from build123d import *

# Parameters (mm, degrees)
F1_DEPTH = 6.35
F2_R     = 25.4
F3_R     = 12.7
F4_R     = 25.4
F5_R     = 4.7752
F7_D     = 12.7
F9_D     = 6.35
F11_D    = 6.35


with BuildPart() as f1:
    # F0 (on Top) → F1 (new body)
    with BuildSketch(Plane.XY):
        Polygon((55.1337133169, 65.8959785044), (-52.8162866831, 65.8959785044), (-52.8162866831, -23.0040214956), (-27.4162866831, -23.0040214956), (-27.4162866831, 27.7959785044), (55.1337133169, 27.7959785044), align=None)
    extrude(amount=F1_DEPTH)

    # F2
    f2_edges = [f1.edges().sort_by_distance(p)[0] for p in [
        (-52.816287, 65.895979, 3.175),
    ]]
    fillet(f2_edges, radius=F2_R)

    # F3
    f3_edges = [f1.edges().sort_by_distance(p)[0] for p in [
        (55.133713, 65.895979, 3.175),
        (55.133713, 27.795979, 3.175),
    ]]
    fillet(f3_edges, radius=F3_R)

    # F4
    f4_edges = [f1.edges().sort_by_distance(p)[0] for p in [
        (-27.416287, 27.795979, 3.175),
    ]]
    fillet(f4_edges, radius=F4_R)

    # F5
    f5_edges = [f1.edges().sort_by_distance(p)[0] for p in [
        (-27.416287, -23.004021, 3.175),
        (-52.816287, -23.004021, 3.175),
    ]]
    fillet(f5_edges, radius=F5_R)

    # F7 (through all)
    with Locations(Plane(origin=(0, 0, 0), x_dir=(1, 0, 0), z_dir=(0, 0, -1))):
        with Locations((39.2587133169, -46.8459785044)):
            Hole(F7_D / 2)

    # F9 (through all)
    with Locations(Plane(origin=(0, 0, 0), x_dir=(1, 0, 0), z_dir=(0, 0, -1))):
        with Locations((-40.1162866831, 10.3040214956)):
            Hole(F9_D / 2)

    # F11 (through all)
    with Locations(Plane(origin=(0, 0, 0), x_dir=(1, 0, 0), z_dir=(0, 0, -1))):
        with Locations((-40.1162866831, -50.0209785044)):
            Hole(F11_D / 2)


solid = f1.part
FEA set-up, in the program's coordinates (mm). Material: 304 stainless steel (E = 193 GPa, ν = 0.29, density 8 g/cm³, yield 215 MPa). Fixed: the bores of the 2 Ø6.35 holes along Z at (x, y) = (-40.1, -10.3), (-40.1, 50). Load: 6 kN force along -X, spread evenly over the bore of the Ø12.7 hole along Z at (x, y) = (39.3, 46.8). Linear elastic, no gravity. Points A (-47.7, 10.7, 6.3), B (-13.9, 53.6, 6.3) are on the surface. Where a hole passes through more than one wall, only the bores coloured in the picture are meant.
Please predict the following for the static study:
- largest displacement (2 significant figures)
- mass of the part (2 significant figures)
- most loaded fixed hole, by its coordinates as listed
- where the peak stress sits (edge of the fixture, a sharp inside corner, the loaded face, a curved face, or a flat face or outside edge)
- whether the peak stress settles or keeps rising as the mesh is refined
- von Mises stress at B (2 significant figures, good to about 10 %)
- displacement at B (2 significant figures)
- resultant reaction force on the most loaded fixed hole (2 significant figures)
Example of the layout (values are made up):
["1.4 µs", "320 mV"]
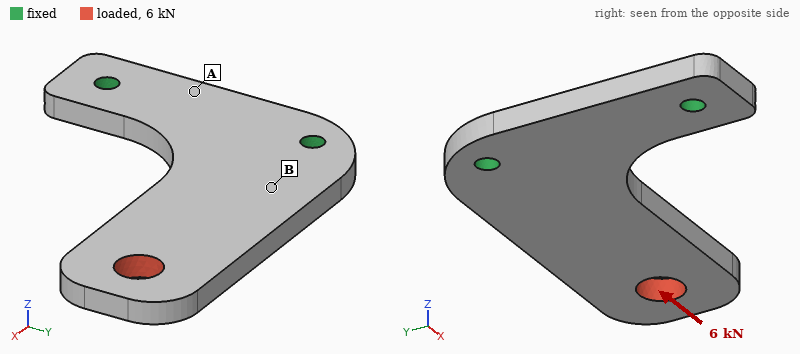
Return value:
["15 µm", "260 g", "(-40.1, 50)", "edge of the fixture", "keeps rising", "27 MPa", "5.1 µm", "5.6 kN"]
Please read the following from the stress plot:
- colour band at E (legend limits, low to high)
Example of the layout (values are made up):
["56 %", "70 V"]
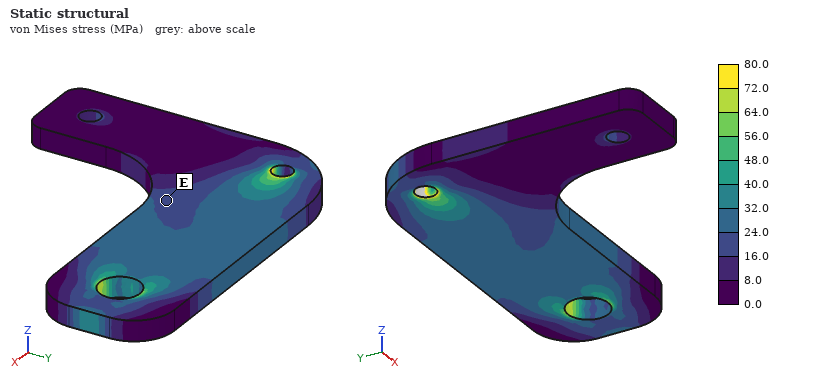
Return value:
["16.0 to 24.0 MPa"]
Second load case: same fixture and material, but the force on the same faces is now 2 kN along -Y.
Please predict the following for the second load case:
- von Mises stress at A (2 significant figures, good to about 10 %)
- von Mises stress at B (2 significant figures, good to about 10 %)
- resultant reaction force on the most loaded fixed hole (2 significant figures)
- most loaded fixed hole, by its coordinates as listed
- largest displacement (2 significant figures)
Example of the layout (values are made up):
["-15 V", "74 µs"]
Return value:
["22 MPa", "27 MPa", "3.1 kN", "(-40.1, -10.3)", "91 µm"]
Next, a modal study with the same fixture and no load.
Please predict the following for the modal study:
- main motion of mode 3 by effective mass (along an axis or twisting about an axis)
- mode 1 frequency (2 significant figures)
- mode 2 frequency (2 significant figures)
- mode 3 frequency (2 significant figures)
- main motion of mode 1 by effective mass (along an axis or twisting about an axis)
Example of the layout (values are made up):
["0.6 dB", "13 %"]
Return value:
["along Y", "630 Hz", "2900 Hz", "3200 Hz", "along Z"]
